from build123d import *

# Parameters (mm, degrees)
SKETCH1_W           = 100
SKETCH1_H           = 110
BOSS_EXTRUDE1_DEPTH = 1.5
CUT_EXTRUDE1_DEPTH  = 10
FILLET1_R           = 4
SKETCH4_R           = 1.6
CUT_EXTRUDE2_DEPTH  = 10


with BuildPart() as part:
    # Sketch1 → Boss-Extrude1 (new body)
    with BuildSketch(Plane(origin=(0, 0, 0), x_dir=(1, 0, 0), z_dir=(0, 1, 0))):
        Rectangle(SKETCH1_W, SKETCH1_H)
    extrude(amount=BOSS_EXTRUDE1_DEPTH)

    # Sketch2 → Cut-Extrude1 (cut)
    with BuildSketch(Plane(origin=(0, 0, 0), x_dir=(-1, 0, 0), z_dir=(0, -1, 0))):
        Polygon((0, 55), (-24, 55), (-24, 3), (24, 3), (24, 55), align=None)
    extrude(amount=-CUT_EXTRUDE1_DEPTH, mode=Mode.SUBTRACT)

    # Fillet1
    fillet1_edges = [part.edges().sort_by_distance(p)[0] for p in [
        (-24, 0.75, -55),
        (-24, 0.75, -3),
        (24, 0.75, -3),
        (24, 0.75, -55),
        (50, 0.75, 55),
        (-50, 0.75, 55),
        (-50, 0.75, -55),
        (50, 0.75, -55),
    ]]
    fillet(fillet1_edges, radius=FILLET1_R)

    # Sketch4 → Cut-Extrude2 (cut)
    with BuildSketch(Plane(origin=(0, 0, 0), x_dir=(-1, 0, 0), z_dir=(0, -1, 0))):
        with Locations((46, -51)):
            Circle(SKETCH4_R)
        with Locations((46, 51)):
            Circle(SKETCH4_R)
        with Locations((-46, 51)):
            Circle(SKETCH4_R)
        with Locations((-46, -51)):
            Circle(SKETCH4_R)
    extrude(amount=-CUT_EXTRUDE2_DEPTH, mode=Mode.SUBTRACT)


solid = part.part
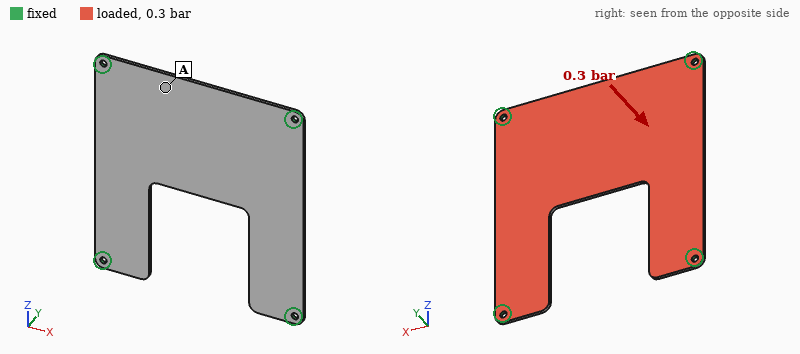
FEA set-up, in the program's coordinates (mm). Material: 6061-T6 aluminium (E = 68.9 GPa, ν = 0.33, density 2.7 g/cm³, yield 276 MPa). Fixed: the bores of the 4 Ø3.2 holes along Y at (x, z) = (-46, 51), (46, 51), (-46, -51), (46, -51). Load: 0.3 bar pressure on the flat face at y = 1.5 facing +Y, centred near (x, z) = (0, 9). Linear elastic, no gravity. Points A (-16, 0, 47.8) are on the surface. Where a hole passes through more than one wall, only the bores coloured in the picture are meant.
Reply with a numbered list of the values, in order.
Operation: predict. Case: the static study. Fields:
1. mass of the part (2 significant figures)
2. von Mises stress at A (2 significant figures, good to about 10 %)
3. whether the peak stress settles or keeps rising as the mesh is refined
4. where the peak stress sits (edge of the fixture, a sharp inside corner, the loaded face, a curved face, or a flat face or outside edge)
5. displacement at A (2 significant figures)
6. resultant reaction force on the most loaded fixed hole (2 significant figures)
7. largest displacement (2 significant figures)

1. 34 g
2. 30 MPa
3. keeps rising
4. edge of the fixture
5. 0.41 mm
6. 75 N
7. 1.3 mm
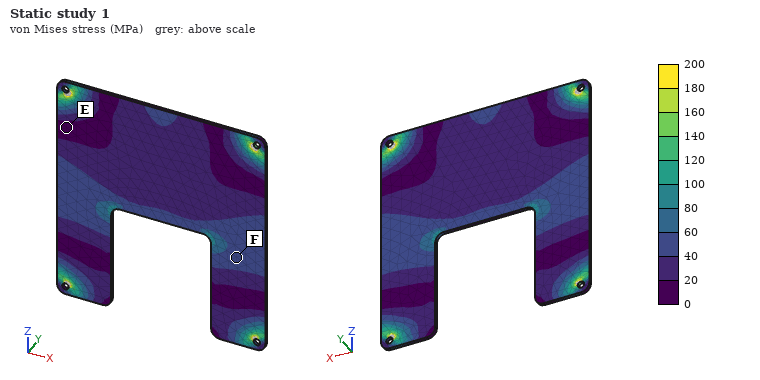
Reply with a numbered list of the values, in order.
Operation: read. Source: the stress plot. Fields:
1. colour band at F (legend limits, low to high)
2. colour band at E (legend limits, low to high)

1. 40 to 60 MPa
2. 0 to 20 MPa
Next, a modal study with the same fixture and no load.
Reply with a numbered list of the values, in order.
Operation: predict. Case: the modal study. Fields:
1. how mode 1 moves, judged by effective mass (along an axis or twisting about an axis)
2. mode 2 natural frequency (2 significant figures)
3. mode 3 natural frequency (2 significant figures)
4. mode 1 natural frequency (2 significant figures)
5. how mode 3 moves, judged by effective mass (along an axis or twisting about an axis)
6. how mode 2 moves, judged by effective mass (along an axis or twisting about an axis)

1. along Y
2. 800 Hz
3. 970 Hz
4. 500 Hz
5. twisting about X
6. twisting about Z
